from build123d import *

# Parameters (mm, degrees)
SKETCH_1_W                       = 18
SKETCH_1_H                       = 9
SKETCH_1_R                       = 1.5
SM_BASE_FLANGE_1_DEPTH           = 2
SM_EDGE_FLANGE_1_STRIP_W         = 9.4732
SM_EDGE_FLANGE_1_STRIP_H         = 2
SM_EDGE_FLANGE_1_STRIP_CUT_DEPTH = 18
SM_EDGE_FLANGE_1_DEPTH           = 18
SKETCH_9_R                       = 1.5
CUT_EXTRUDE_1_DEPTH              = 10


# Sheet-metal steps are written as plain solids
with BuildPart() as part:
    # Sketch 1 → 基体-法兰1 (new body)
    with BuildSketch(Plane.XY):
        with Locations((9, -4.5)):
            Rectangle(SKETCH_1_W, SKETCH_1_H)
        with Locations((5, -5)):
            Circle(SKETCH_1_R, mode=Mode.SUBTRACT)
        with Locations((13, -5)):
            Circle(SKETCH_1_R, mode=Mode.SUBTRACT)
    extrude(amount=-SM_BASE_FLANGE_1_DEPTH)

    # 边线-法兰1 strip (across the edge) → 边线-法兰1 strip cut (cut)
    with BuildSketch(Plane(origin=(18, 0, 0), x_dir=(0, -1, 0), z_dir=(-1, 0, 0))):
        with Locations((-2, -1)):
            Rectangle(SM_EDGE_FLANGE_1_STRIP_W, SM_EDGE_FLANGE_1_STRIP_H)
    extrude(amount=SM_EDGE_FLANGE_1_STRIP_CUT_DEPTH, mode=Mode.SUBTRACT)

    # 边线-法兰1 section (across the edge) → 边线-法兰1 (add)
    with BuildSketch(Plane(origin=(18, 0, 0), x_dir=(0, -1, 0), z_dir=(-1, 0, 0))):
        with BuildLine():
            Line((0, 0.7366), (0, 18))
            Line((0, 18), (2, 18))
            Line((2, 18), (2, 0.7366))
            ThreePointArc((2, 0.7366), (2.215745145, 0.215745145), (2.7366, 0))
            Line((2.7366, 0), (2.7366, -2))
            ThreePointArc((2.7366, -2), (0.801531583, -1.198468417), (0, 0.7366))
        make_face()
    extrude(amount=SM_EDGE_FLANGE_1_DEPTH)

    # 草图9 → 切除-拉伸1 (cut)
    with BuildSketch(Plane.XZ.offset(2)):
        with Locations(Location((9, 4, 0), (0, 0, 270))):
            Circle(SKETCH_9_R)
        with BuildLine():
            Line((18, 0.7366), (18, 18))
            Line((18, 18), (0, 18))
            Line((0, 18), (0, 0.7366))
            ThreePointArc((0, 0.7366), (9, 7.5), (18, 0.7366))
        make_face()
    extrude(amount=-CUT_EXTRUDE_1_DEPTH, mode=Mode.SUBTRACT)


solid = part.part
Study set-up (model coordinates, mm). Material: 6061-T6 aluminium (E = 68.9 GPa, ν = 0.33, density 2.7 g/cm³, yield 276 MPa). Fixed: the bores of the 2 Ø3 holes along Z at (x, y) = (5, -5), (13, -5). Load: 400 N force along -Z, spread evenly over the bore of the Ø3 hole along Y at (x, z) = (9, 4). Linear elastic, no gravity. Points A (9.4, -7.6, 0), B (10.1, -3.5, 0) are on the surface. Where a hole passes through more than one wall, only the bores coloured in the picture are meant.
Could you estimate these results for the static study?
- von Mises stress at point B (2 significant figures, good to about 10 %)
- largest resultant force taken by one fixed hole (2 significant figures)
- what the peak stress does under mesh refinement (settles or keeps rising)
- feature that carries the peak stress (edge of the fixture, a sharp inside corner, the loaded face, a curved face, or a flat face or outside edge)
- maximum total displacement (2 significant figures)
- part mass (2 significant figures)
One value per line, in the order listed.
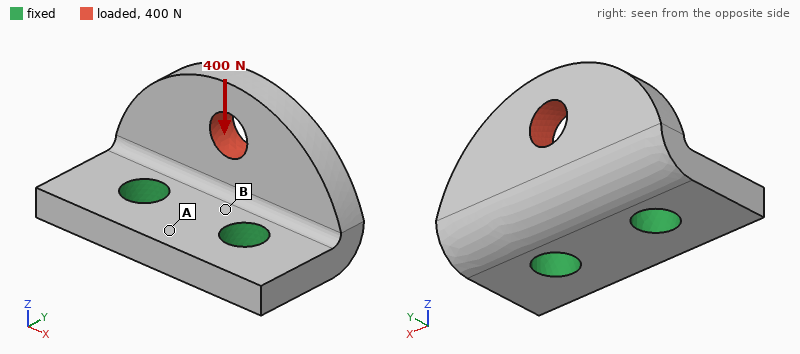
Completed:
50 MPa
200 N
keeps rising
edge of the fixture
28 µm
1.2 g
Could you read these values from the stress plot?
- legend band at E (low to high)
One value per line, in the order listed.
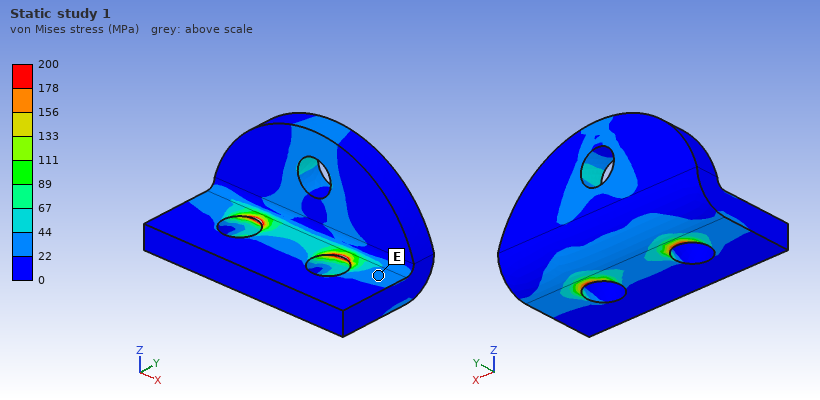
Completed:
22 to 44 MPa
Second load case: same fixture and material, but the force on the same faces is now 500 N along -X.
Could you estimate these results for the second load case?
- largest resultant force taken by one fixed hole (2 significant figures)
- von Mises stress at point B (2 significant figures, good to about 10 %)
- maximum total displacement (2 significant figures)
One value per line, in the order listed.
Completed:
380 N
52 MPa
19 µm
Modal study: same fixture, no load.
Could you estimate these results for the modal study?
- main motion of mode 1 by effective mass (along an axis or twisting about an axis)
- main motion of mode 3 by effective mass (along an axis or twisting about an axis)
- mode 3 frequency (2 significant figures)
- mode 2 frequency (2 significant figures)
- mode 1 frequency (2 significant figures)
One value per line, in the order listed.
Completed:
along Y
along X
52 kHz
33 kHz
20 kHz
